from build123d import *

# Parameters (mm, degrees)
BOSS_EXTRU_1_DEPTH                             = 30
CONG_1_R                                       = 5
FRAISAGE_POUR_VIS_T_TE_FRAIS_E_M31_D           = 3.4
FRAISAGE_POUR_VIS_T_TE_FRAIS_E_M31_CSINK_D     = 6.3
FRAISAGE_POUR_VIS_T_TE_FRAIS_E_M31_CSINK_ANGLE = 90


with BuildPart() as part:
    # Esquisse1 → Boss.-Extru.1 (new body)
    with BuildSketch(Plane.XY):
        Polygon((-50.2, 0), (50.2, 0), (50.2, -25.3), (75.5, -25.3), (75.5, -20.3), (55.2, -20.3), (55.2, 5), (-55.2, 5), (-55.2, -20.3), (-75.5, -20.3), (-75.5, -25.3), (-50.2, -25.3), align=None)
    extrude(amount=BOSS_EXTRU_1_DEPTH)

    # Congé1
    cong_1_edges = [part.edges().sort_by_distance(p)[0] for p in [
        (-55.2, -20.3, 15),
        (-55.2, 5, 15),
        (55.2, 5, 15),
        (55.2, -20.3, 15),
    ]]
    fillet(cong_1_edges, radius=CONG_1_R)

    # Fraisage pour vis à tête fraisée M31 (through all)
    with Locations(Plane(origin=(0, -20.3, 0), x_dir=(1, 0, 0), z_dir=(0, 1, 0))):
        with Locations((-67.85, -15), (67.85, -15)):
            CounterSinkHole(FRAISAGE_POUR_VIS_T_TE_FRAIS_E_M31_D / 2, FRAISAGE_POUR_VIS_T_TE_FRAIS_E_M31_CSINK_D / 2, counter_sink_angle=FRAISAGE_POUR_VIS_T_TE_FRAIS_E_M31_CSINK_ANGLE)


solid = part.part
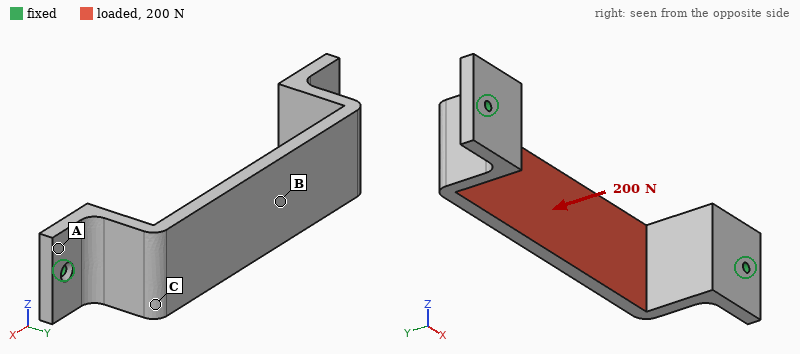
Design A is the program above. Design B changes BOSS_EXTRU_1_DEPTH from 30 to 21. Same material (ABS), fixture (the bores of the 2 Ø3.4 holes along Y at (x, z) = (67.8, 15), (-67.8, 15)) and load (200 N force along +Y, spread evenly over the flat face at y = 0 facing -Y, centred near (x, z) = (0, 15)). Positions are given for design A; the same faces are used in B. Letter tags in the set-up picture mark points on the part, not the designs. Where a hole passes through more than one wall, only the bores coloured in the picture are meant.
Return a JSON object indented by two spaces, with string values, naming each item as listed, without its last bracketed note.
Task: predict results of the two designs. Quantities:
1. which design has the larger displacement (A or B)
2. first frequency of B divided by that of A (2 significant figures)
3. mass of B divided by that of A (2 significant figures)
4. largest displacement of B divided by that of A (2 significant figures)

{
  "which design has the larger displacement": "B",
  "first frequency of B divided by that of A": "1.0",
  "mass of B divided by that of A": "0.70",
  "largest displacement of B divided by that of A": "1.5"
}
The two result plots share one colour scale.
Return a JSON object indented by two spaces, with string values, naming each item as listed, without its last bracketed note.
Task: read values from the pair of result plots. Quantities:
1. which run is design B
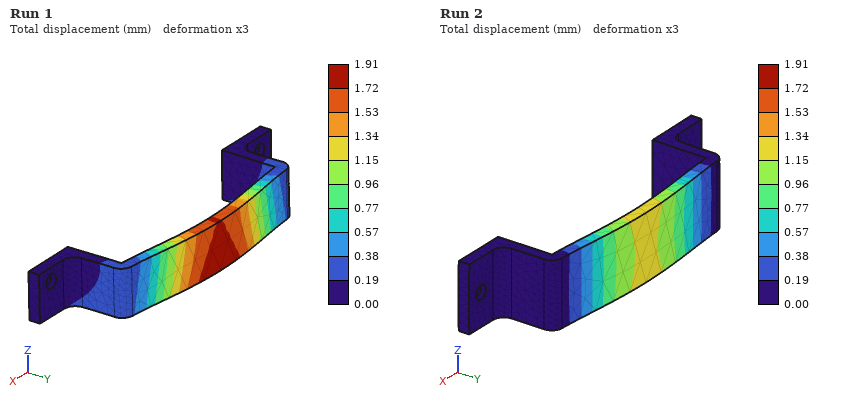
{
  "which run is design B": "Run 1"
}
